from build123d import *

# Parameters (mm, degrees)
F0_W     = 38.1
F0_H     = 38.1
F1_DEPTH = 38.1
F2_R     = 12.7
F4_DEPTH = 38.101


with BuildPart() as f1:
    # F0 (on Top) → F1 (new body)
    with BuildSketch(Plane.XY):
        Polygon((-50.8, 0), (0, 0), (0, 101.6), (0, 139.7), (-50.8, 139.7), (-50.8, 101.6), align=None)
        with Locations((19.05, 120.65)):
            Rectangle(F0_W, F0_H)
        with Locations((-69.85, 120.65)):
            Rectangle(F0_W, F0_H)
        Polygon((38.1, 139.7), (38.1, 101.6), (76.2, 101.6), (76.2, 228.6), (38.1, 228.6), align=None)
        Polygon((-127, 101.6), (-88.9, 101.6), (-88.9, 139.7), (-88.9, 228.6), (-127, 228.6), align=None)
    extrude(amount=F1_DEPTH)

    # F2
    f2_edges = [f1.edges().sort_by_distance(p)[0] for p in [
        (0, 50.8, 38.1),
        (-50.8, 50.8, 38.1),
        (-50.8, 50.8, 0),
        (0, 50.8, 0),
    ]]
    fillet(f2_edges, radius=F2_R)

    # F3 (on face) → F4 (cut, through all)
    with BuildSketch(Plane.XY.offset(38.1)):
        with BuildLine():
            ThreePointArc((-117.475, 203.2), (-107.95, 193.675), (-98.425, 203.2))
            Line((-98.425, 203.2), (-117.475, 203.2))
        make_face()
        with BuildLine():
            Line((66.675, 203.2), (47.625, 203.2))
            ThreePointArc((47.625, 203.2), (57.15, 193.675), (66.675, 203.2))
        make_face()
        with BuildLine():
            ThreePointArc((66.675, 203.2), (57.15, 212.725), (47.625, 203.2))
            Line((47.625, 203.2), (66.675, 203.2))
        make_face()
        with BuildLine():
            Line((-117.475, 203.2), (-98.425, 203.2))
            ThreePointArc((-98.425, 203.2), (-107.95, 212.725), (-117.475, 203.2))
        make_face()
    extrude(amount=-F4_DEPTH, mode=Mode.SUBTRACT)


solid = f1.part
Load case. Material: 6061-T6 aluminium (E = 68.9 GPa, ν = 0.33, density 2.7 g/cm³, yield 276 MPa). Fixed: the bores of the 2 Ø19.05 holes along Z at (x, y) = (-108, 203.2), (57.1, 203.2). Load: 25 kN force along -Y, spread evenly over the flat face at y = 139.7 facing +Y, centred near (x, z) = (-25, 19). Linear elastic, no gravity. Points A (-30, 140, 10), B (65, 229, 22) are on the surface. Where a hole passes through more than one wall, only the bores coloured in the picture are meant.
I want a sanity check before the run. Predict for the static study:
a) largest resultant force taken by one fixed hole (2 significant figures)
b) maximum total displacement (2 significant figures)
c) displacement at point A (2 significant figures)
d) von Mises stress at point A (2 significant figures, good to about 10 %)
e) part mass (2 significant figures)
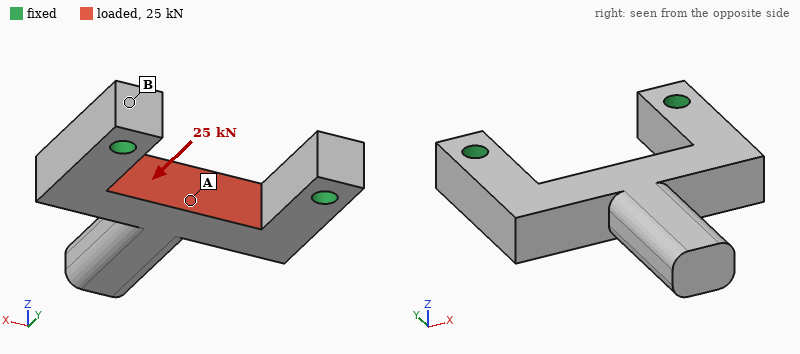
14 kN
57 µm
56 µm
17 MPa
1.9 kg
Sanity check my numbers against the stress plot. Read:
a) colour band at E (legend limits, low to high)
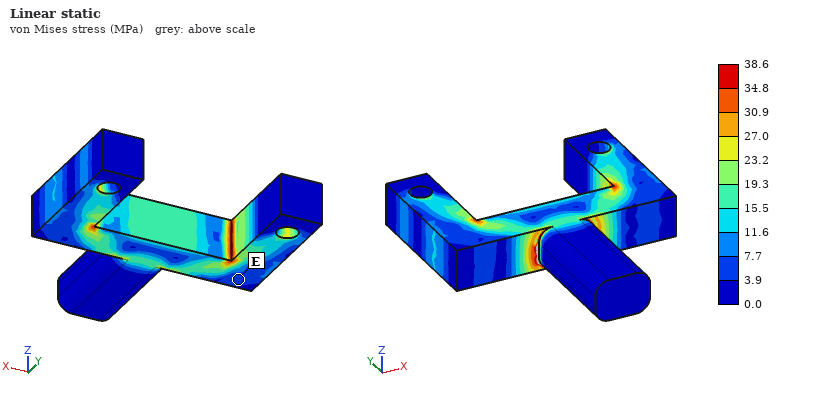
3.9 to 7.7 MPa
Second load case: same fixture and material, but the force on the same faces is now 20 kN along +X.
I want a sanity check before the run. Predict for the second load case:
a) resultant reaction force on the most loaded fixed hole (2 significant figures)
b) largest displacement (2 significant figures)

10 kN
92 µm
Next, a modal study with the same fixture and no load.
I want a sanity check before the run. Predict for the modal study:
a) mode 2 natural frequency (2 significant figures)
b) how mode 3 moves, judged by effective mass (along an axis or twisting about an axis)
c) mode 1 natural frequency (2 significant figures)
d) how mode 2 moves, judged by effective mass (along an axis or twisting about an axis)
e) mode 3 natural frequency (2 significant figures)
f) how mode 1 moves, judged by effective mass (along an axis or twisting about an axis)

2000 Hz
along Z
760 Hz
along X
2600 Hz
along Z
